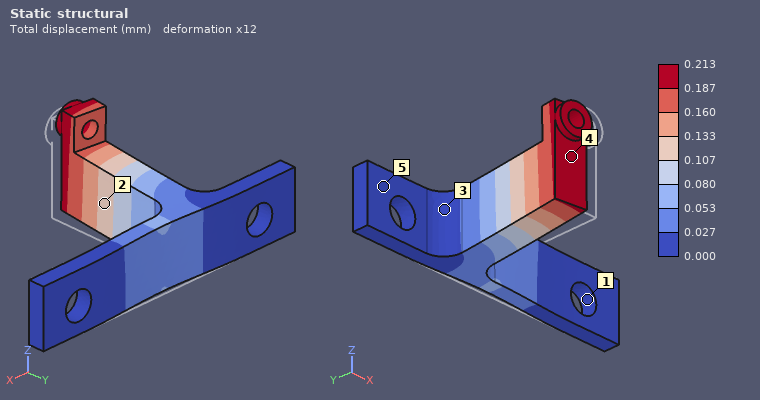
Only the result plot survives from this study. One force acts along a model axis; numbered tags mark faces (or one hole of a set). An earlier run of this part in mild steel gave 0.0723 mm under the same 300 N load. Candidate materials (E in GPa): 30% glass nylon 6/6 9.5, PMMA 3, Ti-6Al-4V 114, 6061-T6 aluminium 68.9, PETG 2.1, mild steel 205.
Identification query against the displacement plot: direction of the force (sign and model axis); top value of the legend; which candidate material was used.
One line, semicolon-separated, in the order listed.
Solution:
-X; 0.213 mm; 6061-T6 aluminium
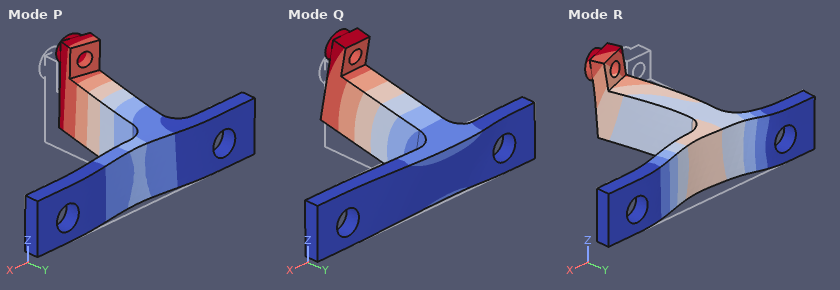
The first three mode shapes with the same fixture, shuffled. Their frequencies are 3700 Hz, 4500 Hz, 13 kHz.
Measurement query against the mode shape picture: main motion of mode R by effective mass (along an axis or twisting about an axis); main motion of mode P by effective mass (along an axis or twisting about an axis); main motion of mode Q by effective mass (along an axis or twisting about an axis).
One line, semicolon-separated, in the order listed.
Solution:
along Y; along X; along Z
